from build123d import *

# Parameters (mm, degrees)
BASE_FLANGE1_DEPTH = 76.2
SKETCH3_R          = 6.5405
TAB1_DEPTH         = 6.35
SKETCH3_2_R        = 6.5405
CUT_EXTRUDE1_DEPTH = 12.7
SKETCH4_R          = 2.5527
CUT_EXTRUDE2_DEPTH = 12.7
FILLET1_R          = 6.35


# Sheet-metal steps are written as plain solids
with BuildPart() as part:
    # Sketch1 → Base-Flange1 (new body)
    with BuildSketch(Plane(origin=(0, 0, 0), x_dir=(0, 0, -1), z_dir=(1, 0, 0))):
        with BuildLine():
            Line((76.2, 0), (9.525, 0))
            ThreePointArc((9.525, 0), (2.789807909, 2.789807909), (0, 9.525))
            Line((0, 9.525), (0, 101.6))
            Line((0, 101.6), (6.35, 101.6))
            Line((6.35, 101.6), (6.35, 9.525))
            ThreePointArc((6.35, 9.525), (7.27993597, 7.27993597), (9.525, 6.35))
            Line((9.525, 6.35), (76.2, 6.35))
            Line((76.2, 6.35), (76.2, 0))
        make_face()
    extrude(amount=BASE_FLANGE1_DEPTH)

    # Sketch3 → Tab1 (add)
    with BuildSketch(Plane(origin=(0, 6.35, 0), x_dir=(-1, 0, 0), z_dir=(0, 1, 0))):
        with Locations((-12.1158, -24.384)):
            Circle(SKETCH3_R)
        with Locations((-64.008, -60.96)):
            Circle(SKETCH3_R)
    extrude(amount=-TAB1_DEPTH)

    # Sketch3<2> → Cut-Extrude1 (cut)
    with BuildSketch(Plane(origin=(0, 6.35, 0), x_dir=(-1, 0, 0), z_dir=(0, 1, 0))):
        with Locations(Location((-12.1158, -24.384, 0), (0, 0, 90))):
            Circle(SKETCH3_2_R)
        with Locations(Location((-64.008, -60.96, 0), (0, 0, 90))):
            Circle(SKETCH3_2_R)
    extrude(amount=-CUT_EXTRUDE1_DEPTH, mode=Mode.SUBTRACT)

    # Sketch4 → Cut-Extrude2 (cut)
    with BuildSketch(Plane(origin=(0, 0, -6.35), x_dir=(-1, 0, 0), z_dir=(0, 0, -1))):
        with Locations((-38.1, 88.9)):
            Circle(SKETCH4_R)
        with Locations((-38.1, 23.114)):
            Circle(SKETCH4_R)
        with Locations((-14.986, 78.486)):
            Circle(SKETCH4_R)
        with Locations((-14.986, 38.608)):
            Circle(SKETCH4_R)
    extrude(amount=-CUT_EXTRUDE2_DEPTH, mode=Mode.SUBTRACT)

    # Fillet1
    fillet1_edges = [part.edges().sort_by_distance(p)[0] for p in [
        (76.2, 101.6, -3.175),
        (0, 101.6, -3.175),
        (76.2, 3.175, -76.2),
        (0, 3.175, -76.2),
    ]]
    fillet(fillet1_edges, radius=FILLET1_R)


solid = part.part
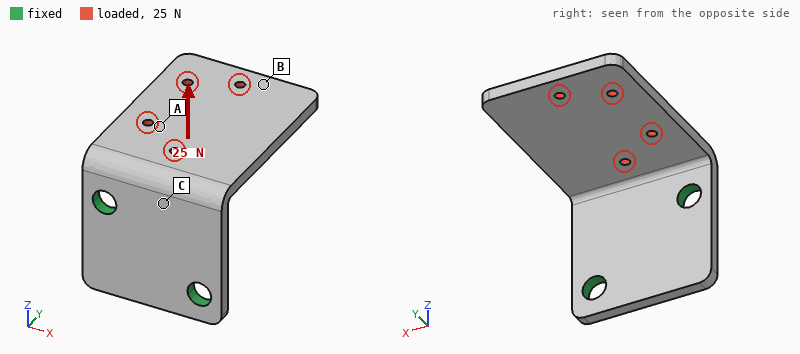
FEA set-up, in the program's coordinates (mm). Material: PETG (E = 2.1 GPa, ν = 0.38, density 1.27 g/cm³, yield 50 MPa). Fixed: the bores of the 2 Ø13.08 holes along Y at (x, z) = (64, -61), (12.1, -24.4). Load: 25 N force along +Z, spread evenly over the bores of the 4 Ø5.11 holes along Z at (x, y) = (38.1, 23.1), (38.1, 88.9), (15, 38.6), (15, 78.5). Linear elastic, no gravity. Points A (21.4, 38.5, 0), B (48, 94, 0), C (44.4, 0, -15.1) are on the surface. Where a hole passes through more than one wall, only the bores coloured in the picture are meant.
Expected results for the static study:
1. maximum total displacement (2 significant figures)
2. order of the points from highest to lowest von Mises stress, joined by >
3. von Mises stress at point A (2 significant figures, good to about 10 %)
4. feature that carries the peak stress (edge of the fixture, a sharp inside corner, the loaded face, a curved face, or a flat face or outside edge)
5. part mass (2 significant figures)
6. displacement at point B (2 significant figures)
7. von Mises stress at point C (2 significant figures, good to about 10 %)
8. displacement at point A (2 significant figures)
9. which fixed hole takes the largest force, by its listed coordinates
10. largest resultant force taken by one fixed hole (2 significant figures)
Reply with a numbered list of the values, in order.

1. 1.7 mm
2. C > A > B
3. 1.1 MPa
4. a flat face or outside edge
5. 100 g
6. 1.5 mm
7. 1.8 MPa
8. 0.49 mm
9. (12.1, -24.4)
10. 20 N
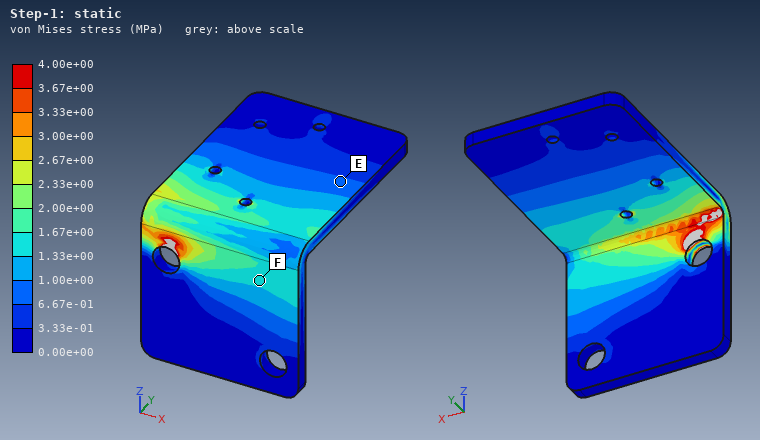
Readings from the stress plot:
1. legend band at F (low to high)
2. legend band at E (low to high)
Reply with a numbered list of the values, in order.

1. 1.33e+00 to 1.67e+00 MPa
2. 6.67e-01 to 1.00e+00 MPa
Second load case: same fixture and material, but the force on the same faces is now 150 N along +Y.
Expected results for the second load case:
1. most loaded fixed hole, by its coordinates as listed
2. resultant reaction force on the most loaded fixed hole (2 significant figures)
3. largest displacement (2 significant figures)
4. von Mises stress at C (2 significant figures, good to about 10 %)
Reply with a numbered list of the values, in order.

1. (12.1, -24.4)
2. 140 N
3. 1.4 mm
4. 1.6 MPa
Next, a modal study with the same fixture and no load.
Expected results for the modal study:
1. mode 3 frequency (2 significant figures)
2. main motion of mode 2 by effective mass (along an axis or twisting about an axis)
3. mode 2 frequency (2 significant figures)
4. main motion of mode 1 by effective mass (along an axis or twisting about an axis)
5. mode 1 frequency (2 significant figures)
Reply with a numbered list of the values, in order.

1. 380 Hz
2. along X
3. 200 Hz
4. along Z
5. 100 Hz
